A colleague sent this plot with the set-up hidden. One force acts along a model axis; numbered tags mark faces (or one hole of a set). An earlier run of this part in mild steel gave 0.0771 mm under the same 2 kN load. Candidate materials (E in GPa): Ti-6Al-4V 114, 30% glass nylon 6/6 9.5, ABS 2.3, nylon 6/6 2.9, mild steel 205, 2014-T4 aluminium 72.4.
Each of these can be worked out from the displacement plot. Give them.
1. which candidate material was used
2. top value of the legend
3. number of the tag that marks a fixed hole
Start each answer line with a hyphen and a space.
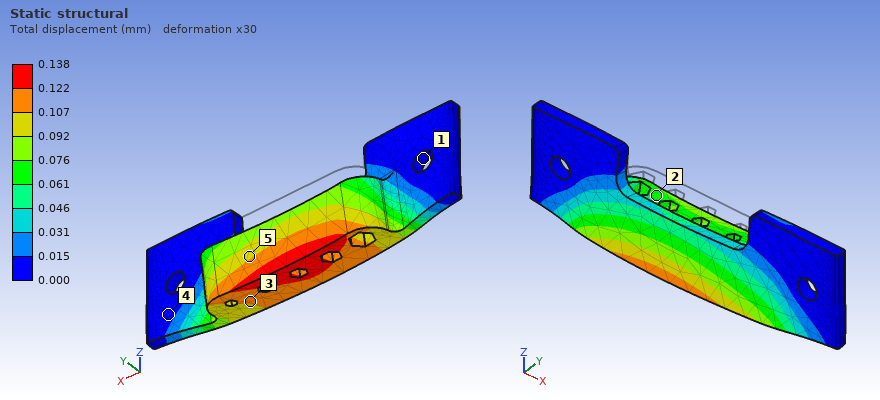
- Ti-6Al-4V
- 0.138 mm
- 1
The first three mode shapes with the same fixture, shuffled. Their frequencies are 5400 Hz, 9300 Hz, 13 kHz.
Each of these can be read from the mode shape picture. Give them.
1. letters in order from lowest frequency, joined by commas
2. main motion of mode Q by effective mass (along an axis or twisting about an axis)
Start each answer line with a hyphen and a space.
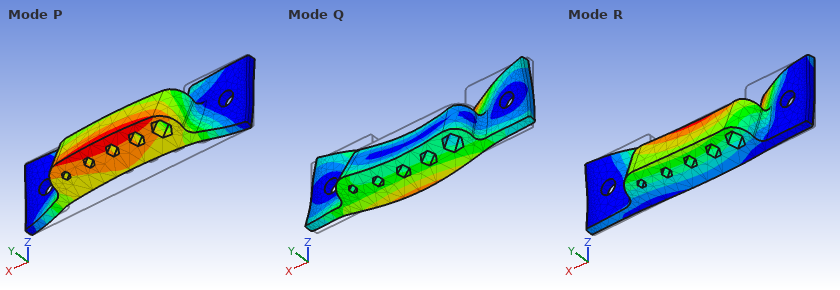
- P, R, Q
- along Z
